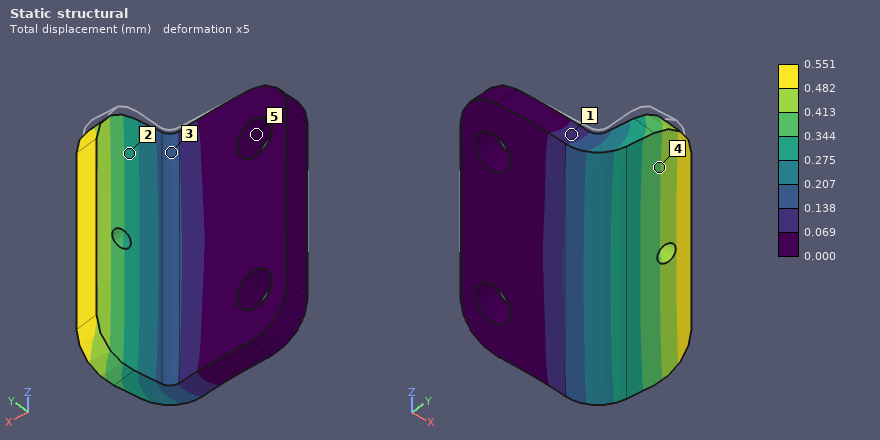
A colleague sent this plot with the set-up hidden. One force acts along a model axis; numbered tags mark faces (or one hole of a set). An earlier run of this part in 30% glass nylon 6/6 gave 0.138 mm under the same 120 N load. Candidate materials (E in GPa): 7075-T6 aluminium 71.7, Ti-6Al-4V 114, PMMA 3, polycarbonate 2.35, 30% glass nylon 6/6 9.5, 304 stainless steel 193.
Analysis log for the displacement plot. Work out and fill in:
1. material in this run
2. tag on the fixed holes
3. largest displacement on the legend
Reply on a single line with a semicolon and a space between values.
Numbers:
polycarbonate; 5; 0.551 mm
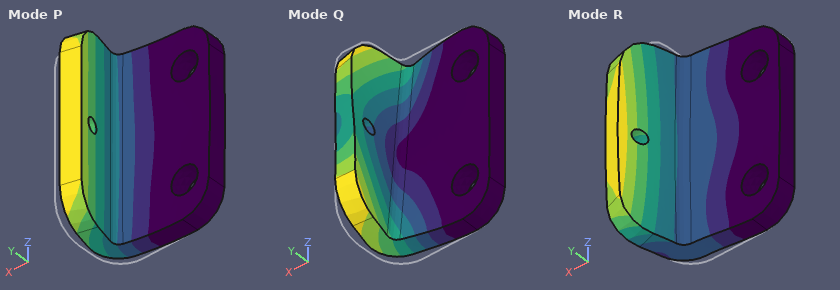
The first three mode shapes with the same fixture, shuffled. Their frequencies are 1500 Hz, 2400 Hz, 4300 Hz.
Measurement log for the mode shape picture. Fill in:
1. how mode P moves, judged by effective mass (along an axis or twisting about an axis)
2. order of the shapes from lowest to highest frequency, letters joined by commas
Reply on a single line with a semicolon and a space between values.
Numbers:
along Y; P, Q, R
